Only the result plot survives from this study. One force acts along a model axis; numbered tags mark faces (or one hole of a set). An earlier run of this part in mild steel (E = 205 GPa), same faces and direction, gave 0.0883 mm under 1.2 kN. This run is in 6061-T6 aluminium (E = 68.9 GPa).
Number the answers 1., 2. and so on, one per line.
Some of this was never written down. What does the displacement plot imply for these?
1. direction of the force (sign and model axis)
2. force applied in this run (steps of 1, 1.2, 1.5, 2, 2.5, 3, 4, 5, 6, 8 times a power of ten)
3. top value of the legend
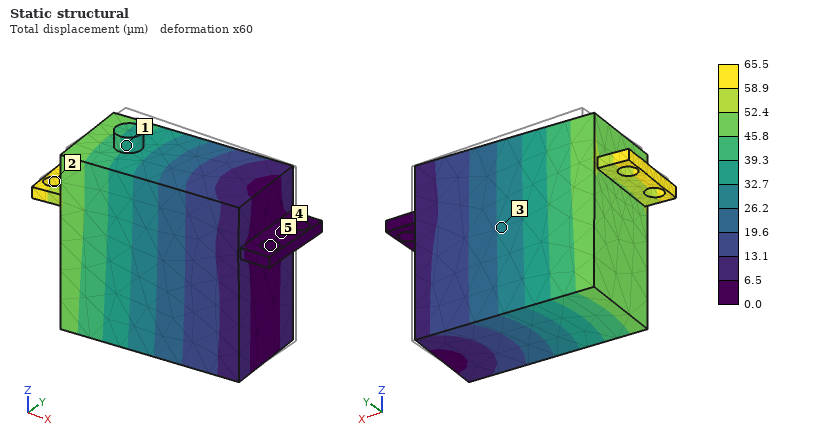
1. -Y
2. 300 N
3. 65.5 µm
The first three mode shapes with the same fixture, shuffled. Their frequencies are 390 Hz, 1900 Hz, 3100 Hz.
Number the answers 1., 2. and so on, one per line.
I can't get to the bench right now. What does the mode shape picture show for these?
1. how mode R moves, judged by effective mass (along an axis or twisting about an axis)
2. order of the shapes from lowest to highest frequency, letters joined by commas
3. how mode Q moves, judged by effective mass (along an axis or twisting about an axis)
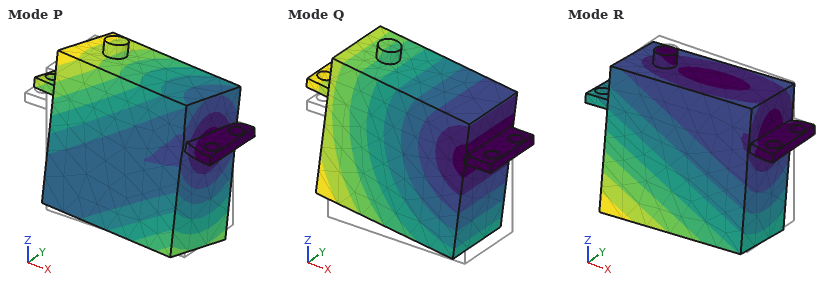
1. along Y
2. Q, R, P
3. along Z
